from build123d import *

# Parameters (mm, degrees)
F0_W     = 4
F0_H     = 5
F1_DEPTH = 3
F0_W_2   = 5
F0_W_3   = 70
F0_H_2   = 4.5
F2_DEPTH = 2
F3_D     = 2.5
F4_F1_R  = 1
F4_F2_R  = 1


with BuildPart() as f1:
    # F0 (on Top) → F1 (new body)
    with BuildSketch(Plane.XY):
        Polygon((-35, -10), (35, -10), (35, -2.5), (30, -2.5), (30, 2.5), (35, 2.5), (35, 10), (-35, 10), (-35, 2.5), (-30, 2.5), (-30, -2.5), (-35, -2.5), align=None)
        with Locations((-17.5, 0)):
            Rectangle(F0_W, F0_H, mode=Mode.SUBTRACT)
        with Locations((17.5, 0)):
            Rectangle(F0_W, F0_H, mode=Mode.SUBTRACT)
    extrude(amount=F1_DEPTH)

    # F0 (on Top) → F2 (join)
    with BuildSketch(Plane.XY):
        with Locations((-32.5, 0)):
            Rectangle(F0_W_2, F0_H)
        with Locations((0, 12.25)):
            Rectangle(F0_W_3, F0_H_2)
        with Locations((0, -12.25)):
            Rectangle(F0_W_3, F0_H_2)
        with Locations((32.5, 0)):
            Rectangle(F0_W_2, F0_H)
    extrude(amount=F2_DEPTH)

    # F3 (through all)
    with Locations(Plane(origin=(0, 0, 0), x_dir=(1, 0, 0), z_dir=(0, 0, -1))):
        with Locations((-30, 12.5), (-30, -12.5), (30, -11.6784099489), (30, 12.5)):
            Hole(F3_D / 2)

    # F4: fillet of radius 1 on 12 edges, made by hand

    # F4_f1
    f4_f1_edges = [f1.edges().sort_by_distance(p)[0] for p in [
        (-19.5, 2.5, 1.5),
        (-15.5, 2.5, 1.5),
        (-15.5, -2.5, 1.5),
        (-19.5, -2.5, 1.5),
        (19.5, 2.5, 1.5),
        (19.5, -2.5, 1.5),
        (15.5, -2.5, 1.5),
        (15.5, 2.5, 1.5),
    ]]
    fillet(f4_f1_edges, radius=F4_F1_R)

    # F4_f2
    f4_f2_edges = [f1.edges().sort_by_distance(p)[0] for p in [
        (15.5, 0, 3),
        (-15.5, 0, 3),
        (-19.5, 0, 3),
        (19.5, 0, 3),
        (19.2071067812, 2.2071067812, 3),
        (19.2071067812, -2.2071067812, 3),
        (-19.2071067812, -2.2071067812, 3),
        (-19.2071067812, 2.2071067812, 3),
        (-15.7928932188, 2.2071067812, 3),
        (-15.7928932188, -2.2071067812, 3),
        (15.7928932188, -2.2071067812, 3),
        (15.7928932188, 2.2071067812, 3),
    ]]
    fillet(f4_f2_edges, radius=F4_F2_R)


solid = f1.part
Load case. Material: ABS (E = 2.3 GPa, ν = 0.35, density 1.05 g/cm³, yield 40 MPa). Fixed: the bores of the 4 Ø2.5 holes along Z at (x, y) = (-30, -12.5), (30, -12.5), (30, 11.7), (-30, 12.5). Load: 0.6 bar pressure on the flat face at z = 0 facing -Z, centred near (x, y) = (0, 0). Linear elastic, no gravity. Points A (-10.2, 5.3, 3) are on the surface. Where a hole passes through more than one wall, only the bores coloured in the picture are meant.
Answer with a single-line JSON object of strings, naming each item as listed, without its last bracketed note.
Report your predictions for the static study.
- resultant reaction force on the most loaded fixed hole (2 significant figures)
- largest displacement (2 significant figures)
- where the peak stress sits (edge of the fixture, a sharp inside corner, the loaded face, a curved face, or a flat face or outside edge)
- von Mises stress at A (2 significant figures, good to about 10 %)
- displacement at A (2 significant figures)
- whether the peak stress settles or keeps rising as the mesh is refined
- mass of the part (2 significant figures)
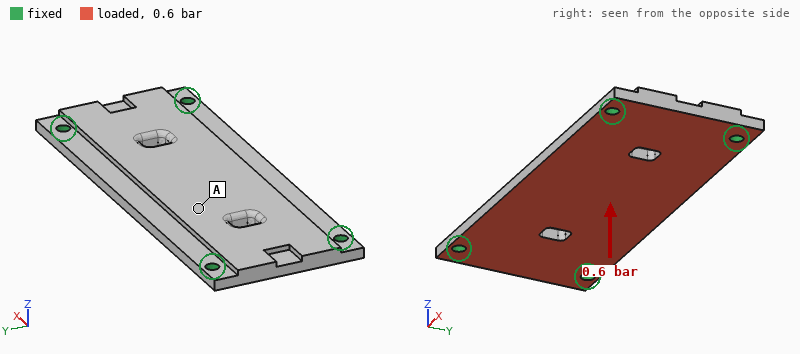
{"resultant reaction force on the most loaded fixed hole": "40 N", "largest displacement": "0.81 mm", "where the peak stress sits": "edge of the fixture", "von Mises stress at A": "7.4 MPa", "displacement at A": "0.62 mm", "whether the peak stress settles or keeps rising as the mesh is refined": "keeps rising", "mass of the part": "5.5 g"}
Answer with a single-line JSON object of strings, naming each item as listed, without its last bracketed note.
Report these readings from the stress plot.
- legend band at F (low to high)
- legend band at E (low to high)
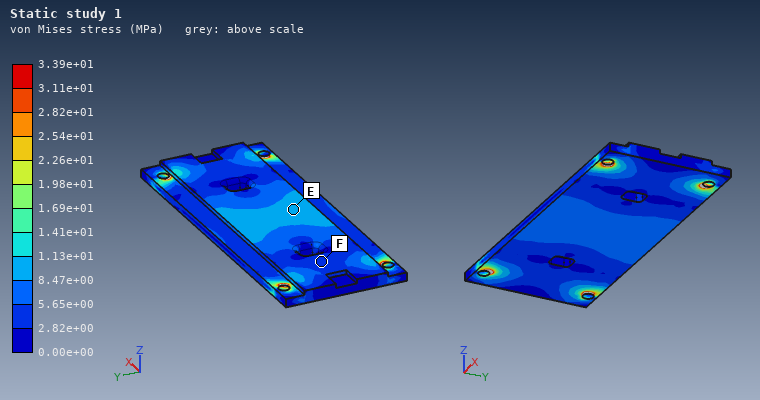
{"legend band at F": "2.82e+00 to 5.65e+00 MPa", "legend band at E": "8.47e+00 to 1.13e+01 MPa"}
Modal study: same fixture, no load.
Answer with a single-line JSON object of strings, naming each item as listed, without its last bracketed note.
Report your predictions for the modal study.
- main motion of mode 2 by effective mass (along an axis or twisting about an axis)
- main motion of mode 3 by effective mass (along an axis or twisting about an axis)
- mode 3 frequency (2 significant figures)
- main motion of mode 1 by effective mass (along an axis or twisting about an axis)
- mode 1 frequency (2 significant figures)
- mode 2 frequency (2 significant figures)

{"main motion of mode 2 by effective mass": "twisting about X", "main motion of mode 3 by effective mass": "twisting about Y", "mode 3 frequency": "2600 Hz", "main motion of mode 1 by effective mass": "along Z", "mode 1 frequency": "950 Hz", "mode 2 frequency": "1800 Hz"}
